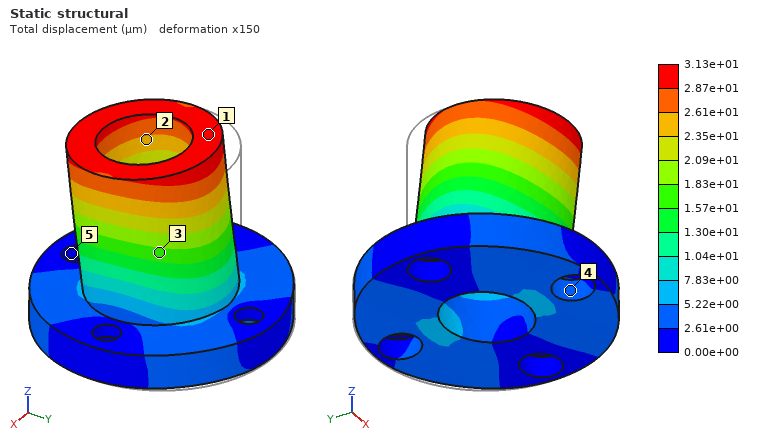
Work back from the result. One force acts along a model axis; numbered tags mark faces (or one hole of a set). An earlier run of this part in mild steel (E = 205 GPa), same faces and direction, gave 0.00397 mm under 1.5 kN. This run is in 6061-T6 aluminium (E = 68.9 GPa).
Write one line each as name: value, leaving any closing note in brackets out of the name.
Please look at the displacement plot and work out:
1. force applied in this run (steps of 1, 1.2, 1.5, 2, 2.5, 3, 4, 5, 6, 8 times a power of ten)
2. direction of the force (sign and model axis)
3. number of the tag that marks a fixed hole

force applied in this run: 4 kN
direction of the force: -Y
number of the tag that marks a fixed hole: 5
